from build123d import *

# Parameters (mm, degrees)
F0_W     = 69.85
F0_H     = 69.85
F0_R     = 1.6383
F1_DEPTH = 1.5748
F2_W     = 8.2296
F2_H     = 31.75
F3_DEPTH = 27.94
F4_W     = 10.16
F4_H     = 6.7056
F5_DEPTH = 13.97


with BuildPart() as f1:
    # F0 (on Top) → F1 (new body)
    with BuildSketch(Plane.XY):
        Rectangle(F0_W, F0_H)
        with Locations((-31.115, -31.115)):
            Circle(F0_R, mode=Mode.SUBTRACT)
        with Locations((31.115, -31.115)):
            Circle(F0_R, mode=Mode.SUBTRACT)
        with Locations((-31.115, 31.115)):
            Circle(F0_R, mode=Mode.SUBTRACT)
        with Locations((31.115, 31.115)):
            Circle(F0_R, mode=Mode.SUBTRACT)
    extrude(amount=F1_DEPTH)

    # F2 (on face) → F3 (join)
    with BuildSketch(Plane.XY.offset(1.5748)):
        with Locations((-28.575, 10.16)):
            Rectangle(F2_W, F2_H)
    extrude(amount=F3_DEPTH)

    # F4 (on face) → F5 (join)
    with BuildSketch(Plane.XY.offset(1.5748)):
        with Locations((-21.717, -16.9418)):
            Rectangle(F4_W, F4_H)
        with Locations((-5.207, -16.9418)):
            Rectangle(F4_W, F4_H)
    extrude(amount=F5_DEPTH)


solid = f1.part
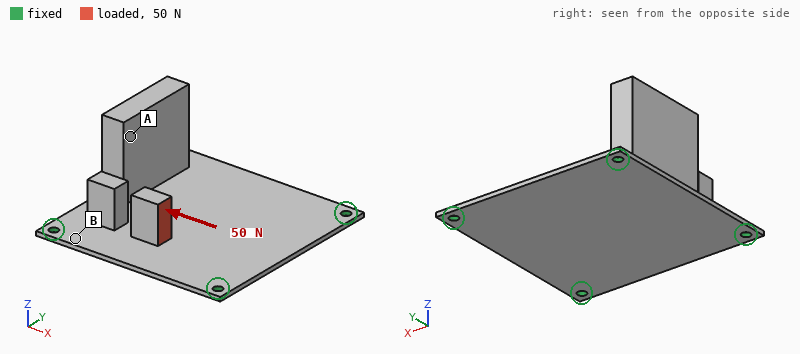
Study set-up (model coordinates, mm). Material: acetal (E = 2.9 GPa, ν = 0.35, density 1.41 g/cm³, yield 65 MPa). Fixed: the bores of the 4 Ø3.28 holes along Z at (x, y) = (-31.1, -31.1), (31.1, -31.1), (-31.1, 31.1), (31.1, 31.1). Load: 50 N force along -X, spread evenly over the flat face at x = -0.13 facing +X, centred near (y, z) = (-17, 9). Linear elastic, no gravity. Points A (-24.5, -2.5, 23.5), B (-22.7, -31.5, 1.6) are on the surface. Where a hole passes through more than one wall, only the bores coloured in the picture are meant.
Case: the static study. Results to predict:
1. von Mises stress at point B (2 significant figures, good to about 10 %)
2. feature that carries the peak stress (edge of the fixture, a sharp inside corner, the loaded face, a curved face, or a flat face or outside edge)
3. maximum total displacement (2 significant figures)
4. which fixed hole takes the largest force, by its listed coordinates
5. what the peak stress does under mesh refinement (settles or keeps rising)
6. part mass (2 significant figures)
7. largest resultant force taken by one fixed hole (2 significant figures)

3.1 MPa
edge of the fixture
0.67 mm
(-31.1, -31.1)
keeps rising
24 g
22 N
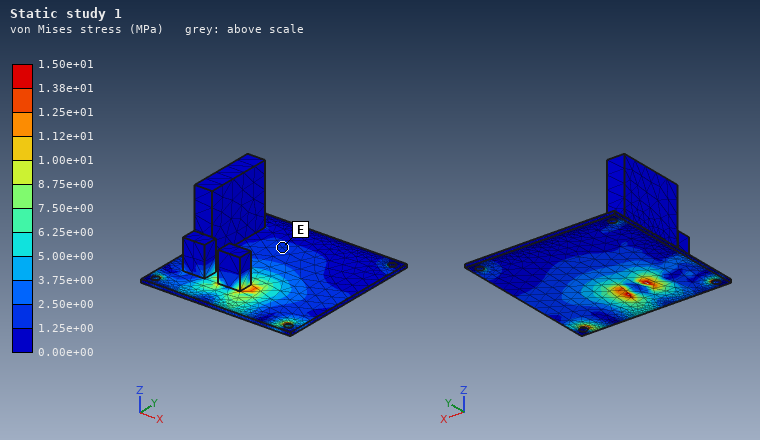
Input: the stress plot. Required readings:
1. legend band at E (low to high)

1.25e+00 to 2.50e+00 MPa
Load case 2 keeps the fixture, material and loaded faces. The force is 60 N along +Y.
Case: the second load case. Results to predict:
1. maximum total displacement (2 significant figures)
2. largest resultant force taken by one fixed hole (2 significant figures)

1.0 mm
22 N
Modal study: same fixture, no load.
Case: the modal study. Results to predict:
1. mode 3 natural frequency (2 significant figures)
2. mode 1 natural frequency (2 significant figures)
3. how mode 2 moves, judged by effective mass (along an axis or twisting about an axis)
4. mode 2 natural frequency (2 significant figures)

530 Hz
260 Hz
along Z
300 Hz
